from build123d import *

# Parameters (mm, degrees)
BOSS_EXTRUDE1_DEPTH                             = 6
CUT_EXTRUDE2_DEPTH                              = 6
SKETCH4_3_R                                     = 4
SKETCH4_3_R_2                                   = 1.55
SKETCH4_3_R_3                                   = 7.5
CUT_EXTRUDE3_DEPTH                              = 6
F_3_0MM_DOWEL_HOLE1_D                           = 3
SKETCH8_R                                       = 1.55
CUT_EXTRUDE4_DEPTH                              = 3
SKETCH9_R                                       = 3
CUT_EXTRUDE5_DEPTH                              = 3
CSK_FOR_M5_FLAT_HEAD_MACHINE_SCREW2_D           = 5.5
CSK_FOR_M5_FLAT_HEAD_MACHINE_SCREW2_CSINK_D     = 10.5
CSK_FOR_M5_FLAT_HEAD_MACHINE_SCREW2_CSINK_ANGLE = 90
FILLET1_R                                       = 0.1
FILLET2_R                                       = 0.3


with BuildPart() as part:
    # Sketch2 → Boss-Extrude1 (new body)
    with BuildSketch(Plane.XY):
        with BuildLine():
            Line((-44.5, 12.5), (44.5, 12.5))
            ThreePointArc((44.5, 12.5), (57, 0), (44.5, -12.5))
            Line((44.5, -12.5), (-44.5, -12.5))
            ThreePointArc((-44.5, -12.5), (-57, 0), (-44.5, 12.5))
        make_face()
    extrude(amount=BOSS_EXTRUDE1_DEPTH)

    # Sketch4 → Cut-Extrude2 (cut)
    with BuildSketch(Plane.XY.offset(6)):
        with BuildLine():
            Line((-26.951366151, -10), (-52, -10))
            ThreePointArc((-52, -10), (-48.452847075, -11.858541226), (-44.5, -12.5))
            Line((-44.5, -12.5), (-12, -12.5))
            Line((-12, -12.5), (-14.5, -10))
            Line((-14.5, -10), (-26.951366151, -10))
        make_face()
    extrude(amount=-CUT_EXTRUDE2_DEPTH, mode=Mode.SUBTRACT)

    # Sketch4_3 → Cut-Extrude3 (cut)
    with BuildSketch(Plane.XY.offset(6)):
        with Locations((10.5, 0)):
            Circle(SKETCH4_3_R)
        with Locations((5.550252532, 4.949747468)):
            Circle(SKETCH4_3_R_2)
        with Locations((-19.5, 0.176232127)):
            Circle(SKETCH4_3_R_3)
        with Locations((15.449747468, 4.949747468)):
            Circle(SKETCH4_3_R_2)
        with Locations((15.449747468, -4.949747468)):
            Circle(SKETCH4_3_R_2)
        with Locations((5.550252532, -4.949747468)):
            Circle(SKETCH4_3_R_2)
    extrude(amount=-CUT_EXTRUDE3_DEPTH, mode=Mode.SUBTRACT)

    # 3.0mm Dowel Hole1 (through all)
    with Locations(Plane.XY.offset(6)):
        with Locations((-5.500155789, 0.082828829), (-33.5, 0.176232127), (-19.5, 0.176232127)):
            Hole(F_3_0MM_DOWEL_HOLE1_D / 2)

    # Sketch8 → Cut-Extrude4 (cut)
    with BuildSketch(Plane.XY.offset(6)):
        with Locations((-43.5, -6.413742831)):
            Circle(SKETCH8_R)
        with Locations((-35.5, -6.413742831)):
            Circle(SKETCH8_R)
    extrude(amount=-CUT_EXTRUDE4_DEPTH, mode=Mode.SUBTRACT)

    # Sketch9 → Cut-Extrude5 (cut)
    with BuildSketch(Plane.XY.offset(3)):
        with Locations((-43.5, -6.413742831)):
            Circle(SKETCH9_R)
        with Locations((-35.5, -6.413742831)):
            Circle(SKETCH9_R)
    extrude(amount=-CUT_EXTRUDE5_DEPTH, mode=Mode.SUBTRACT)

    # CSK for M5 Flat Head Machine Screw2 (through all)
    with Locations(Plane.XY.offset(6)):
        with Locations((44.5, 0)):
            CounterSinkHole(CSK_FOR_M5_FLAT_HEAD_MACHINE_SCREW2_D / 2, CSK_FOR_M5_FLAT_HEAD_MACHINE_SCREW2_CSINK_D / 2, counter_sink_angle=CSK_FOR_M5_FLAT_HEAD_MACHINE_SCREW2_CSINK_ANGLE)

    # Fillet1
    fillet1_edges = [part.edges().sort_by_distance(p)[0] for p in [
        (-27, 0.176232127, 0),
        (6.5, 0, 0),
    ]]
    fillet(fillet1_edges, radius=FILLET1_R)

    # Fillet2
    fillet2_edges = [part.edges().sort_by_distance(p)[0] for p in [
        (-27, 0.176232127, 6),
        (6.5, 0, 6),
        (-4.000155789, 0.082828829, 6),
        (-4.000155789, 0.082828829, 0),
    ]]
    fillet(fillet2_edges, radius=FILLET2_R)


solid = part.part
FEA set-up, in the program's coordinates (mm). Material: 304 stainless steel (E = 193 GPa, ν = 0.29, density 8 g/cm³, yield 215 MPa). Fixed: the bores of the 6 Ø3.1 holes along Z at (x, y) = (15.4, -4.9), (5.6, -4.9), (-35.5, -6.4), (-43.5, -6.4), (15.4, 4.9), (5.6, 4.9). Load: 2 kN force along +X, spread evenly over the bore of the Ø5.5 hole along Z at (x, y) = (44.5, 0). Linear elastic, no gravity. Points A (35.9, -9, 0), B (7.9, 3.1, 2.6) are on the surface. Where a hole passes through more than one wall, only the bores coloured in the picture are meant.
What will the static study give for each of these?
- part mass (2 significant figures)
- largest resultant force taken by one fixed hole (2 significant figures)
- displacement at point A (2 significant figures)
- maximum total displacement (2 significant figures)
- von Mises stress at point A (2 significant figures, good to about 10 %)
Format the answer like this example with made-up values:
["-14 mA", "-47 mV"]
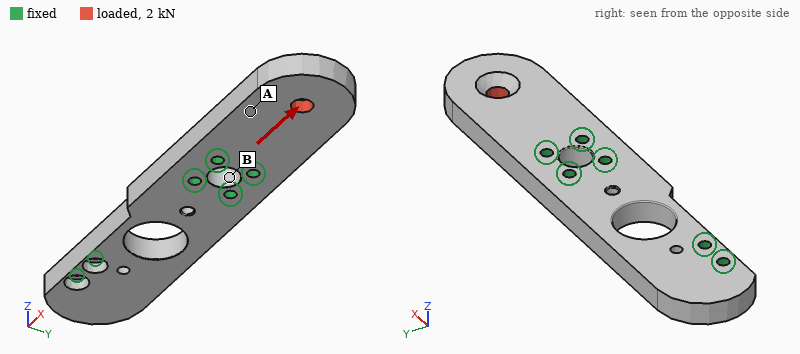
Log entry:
["110 g", "880 N", "6.8 µm", "23 µm", "27 MPa"]
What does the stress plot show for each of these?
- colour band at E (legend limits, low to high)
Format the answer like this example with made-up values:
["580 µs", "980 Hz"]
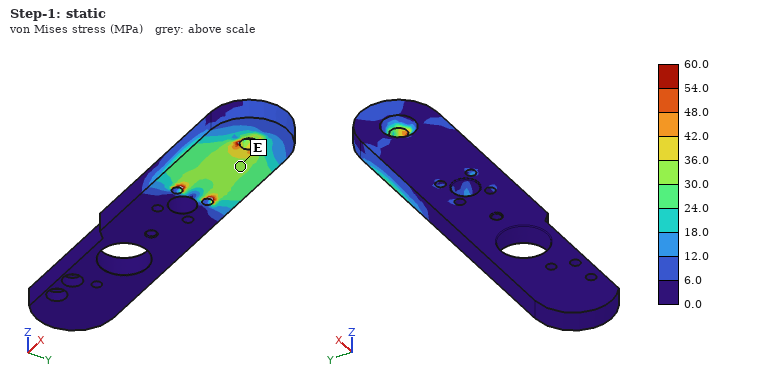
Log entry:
["30.0 to 36.0 MPa"]
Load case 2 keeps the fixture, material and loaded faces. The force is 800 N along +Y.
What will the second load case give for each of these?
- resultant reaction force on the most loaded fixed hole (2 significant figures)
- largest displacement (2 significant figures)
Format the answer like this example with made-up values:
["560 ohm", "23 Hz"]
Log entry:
["1.3 kN", "13 µm"]
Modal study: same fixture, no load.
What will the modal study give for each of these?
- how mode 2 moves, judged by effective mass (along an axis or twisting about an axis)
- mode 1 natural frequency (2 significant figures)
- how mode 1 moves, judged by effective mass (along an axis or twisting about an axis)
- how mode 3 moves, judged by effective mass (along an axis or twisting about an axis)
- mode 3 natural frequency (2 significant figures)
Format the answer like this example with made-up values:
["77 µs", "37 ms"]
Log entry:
["along Z", "3100 Hz", "along Z", "along Y", "9300 Hz"]
